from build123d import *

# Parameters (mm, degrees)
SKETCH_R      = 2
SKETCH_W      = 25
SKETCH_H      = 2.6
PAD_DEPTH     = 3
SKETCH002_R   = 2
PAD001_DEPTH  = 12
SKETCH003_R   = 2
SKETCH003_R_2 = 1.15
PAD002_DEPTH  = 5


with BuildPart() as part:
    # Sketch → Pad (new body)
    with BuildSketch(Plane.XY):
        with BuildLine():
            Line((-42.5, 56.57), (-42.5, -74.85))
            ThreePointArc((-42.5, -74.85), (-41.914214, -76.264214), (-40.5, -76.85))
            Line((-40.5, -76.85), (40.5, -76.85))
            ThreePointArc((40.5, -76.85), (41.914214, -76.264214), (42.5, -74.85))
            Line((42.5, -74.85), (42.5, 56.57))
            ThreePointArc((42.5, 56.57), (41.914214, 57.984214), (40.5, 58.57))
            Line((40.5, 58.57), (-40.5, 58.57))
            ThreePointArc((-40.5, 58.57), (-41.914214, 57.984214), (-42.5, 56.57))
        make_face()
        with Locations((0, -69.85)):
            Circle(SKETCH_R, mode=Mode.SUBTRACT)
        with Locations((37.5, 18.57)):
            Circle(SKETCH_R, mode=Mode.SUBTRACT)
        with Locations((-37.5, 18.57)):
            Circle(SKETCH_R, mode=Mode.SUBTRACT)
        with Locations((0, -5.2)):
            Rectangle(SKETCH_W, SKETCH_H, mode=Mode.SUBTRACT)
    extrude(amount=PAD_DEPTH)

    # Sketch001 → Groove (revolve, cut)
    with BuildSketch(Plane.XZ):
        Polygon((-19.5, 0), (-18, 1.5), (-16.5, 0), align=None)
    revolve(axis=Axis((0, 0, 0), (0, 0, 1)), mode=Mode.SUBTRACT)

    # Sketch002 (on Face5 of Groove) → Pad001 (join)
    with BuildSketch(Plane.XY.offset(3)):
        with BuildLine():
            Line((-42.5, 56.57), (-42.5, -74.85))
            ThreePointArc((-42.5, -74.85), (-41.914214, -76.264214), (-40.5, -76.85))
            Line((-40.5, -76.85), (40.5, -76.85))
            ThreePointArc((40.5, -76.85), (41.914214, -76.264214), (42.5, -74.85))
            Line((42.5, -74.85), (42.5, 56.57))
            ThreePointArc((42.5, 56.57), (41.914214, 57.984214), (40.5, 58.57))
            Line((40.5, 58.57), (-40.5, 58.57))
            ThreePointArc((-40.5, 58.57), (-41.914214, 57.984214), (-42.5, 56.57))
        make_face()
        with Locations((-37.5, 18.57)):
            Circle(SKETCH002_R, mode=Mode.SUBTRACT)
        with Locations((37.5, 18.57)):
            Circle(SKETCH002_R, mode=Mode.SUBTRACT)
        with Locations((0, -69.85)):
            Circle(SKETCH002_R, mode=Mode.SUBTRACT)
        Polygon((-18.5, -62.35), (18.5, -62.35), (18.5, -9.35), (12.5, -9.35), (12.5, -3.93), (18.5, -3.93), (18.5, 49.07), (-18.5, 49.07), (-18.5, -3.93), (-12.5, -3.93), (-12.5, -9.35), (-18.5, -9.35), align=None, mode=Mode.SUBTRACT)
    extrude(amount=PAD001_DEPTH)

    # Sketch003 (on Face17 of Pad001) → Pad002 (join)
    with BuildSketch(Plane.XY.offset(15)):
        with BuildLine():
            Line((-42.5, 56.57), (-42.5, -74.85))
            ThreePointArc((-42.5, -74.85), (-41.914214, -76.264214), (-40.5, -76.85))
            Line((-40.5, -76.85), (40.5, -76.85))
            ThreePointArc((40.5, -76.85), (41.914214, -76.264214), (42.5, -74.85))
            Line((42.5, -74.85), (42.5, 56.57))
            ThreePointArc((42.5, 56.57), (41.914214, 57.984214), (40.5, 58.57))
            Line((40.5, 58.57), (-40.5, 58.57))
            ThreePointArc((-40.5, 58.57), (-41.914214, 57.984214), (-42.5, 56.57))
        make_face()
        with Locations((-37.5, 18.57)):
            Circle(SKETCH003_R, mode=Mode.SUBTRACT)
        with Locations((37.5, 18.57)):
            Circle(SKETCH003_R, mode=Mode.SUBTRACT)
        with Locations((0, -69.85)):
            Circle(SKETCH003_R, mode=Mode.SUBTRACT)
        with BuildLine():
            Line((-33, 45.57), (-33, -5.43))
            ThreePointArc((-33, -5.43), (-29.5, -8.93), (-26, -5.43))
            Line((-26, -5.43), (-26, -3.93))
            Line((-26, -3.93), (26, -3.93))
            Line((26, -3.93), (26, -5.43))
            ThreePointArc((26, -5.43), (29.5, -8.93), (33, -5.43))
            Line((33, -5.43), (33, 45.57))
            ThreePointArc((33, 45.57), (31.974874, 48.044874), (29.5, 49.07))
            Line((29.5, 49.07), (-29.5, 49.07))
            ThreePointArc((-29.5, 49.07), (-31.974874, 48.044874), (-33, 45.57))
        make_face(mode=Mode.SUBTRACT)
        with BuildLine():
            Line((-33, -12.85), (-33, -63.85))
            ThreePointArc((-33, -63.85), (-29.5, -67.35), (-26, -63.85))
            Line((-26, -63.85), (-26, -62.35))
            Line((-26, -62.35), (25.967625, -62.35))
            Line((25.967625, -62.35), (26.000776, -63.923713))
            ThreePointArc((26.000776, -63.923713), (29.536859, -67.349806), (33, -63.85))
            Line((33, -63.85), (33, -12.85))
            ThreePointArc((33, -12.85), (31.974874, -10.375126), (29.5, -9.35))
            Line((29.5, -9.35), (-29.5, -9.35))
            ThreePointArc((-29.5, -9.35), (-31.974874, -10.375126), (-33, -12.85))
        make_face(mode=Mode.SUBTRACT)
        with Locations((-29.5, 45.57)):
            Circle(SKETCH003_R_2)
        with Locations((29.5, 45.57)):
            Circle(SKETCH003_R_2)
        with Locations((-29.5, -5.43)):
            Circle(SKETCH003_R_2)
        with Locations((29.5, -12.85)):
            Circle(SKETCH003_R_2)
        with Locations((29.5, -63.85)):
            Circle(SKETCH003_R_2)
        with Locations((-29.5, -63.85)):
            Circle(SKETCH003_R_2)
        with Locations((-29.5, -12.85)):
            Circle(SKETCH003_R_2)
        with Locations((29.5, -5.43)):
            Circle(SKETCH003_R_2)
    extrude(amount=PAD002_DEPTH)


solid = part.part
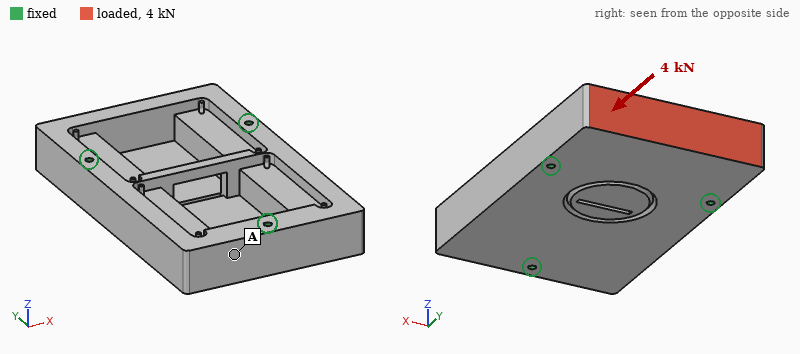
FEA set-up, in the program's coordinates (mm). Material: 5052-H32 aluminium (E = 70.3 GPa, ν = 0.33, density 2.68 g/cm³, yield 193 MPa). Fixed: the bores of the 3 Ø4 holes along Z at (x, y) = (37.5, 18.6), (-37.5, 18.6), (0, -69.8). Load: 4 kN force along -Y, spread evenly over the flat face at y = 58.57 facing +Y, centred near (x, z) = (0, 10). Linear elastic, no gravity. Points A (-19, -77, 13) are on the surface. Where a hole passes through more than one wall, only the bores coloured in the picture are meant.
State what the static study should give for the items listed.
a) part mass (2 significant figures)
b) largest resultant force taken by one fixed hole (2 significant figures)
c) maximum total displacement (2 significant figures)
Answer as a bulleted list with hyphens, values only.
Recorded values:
- 390 g
- 2.0 kN
- 18 µm
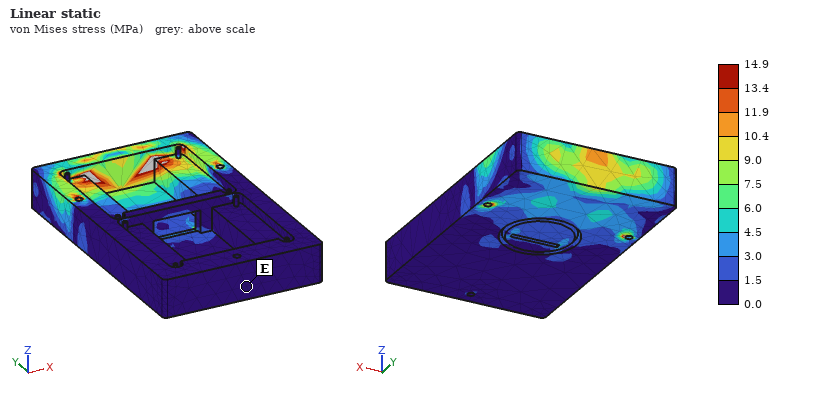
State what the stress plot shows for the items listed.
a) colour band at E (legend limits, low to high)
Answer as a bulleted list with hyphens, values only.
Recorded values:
- 0.0 to 1.5 MPa
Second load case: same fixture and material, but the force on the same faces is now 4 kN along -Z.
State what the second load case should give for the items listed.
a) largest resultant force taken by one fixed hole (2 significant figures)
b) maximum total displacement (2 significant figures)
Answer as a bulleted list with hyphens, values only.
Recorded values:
- 2.2 kN
- 98 µm
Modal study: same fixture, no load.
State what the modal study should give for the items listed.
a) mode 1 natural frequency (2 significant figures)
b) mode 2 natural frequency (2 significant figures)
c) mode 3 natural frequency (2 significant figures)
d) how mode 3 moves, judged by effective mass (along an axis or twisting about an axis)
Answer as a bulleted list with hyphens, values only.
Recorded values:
- 5200 Hz
- 5300 Hz
- 5800 Hz
- along Z
